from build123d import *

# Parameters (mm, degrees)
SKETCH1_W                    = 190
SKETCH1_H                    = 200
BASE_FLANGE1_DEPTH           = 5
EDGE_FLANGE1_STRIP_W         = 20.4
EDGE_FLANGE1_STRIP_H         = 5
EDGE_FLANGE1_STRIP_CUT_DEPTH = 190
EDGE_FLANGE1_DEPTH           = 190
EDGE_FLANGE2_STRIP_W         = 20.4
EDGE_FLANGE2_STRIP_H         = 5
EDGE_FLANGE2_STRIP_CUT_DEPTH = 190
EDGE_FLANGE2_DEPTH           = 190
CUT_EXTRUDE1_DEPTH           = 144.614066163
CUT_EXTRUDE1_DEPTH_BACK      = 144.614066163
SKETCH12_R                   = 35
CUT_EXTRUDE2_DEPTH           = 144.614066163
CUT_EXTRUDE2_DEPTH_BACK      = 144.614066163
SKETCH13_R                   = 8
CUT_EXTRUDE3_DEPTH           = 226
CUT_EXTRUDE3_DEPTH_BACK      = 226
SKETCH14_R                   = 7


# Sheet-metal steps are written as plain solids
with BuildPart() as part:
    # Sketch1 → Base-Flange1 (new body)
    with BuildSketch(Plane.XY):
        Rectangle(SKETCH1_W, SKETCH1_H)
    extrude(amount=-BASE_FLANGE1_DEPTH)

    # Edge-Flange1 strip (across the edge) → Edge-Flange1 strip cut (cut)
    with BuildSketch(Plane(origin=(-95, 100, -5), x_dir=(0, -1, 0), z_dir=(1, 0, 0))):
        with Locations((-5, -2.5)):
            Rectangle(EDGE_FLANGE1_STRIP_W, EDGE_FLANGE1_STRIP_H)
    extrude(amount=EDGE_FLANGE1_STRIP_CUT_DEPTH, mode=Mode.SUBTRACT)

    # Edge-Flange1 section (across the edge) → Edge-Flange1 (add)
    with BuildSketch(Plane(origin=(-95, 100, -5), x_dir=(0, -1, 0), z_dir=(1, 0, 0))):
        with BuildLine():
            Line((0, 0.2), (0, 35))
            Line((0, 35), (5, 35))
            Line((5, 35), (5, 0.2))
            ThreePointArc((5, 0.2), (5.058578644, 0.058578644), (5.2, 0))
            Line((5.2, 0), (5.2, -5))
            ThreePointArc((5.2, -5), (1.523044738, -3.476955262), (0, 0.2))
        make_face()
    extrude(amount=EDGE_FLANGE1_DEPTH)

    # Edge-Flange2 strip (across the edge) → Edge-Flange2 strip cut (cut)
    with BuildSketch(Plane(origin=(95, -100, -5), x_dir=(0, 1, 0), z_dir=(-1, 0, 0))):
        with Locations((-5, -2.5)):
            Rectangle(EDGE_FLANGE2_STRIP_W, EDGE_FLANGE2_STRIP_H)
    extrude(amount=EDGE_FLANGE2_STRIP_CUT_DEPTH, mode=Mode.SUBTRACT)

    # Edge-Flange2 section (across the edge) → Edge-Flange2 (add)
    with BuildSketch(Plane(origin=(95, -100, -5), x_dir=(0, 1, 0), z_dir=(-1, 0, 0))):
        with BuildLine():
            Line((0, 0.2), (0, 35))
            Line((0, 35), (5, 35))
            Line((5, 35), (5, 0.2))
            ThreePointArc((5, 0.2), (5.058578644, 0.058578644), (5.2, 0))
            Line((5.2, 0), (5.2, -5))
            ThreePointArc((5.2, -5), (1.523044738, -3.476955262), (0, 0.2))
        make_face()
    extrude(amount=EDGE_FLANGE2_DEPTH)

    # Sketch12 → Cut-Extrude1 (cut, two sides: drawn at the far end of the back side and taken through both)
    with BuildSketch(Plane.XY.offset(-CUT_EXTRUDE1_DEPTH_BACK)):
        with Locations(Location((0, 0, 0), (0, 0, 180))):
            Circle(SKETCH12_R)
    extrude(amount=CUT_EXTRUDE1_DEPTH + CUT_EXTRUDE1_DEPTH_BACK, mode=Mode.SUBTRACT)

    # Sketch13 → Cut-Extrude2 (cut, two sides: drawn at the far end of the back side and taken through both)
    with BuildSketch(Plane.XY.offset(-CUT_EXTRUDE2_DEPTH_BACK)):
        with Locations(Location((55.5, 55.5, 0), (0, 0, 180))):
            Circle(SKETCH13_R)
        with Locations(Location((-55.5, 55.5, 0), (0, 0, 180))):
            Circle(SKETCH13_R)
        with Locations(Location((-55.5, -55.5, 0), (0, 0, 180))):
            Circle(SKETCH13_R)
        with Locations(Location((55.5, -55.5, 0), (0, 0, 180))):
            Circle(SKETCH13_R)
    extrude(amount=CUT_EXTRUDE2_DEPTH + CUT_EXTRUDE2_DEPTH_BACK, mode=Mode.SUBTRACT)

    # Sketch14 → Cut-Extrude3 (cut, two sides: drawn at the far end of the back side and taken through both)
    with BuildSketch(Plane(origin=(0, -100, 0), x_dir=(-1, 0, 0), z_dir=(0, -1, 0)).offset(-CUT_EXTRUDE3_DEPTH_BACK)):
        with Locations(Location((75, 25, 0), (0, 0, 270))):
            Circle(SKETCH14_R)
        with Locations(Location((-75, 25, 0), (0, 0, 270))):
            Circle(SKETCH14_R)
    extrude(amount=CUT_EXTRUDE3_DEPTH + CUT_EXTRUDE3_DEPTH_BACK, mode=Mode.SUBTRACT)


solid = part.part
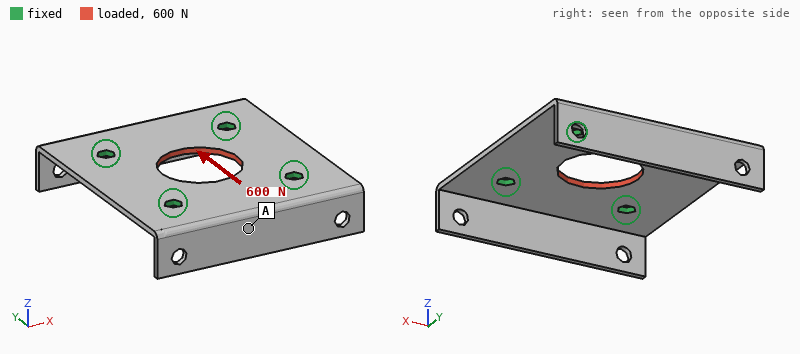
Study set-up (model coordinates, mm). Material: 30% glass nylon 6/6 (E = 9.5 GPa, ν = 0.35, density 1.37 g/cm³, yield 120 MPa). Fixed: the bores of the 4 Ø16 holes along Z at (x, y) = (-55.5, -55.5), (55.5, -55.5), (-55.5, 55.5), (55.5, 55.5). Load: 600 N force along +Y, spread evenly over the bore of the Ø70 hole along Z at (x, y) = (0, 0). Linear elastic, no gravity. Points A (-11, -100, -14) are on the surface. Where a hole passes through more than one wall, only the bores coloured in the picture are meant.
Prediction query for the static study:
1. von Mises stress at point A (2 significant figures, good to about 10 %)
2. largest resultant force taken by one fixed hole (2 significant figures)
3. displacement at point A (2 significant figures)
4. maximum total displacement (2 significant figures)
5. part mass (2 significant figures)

0.18 MPa
150 N
3.4 µm
4.9 µm
310 g
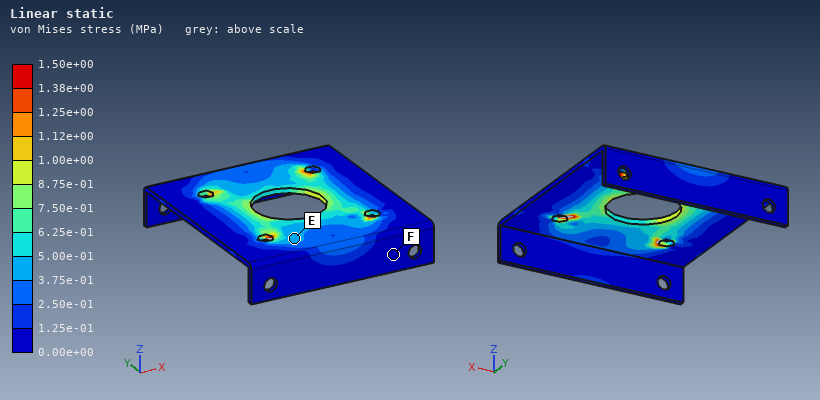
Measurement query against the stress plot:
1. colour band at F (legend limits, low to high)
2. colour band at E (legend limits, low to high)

0.00e+00 to 1.25e-01 MPa
3.75e-01 to 5.00e-01 MPa
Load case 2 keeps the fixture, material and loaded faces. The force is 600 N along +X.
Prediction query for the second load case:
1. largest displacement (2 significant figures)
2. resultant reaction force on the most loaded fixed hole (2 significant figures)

5.2 µm
160 N
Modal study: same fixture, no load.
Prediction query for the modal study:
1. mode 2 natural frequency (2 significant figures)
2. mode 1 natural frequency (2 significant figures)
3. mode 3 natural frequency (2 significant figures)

490 Hz
490 Hz
640 Hz
